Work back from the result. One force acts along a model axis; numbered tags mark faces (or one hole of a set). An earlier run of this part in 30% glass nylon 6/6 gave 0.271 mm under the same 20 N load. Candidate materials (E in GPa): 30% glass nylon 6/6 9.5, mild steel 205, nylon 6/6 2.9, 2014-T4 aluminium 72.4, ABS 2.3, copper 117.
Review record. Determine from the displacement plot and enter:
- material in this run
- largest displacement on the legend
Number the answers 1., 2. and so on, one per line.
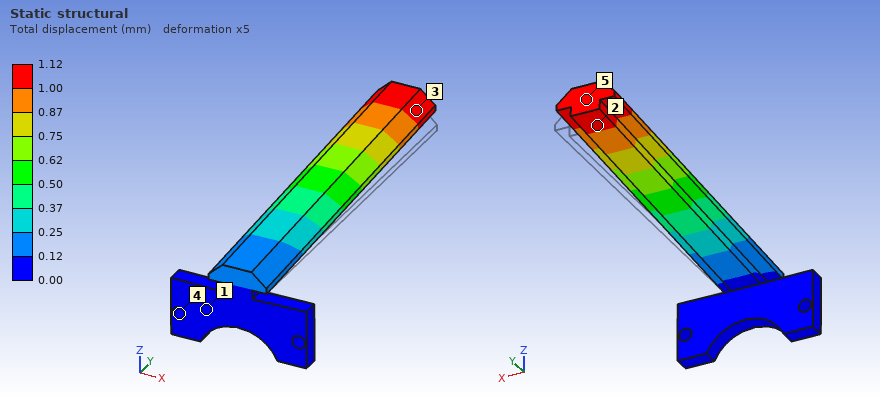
1. ABS
2. 1.12 mm
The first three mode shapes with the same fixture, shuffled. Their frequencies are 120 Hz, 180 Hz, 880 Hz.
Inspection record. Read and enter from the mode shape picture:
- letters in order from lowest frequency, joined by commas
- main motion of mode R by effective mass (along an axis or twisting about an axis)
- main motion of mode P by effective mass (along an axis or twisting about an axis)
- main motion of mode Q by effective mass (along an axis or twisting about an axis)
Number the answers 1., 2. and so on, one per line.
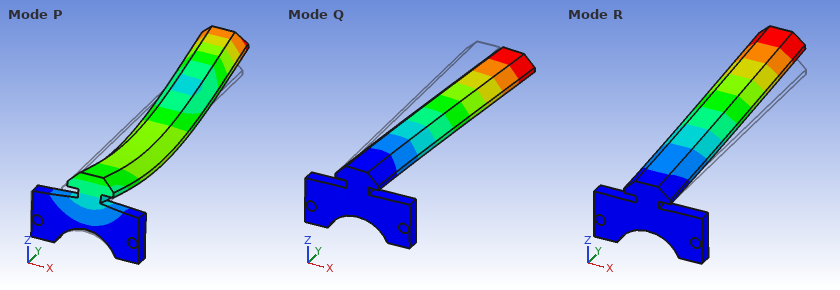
1. R, Q, P
2. along Z
3. along Y
4. along X
